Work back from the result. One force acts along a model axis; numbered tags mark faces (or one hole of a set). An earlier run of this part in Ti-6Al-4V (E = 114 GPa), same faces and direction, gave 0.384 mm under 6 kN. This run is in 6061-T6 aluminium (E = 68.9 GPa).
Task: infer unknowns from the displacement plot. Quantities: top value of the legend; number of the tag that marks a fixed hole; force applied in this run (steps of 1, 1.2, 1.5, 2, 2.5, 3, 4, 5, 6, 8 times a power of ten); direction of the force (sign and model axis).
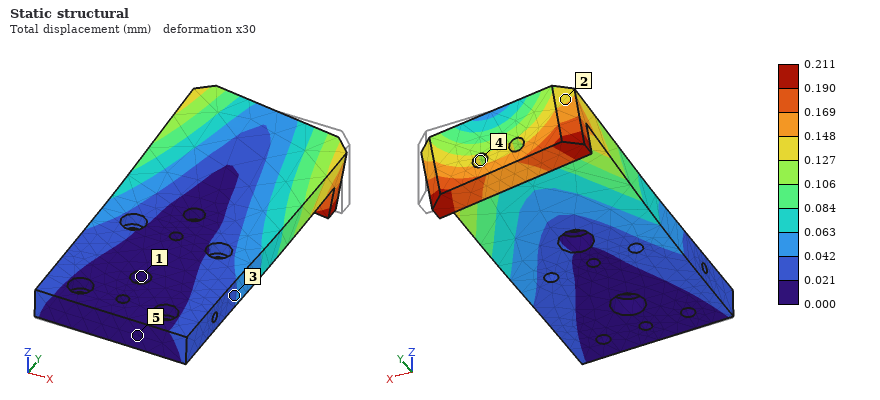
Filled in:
0.211 mm
1
2 kN
-X
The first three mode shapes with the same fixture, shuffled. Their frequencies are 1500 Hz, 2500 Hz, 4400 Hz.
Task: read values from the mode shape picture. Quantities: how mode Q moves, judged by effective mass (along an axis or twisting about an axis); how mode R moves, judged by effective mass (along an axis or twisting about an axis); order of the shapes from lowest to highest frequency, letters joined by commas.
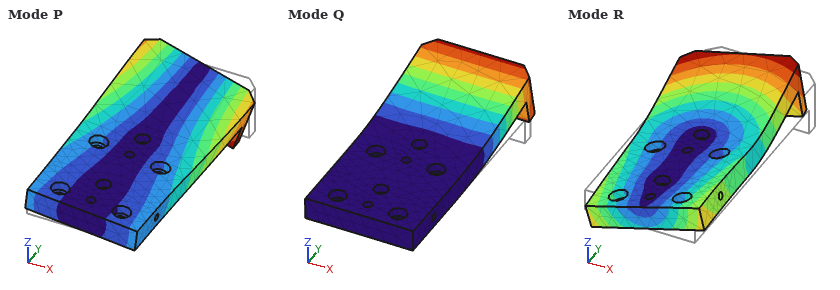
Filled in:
along Z
along X
Q, P, R
